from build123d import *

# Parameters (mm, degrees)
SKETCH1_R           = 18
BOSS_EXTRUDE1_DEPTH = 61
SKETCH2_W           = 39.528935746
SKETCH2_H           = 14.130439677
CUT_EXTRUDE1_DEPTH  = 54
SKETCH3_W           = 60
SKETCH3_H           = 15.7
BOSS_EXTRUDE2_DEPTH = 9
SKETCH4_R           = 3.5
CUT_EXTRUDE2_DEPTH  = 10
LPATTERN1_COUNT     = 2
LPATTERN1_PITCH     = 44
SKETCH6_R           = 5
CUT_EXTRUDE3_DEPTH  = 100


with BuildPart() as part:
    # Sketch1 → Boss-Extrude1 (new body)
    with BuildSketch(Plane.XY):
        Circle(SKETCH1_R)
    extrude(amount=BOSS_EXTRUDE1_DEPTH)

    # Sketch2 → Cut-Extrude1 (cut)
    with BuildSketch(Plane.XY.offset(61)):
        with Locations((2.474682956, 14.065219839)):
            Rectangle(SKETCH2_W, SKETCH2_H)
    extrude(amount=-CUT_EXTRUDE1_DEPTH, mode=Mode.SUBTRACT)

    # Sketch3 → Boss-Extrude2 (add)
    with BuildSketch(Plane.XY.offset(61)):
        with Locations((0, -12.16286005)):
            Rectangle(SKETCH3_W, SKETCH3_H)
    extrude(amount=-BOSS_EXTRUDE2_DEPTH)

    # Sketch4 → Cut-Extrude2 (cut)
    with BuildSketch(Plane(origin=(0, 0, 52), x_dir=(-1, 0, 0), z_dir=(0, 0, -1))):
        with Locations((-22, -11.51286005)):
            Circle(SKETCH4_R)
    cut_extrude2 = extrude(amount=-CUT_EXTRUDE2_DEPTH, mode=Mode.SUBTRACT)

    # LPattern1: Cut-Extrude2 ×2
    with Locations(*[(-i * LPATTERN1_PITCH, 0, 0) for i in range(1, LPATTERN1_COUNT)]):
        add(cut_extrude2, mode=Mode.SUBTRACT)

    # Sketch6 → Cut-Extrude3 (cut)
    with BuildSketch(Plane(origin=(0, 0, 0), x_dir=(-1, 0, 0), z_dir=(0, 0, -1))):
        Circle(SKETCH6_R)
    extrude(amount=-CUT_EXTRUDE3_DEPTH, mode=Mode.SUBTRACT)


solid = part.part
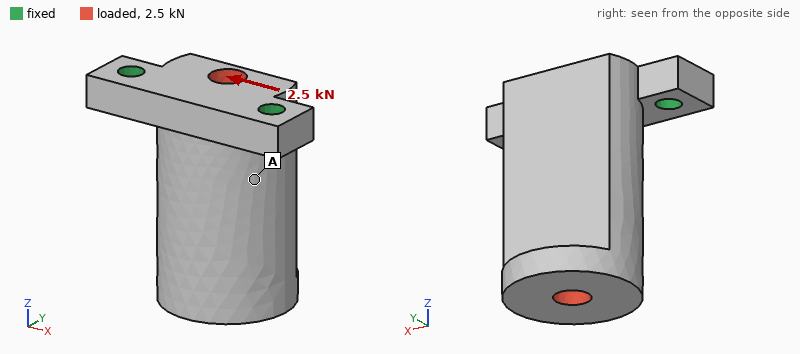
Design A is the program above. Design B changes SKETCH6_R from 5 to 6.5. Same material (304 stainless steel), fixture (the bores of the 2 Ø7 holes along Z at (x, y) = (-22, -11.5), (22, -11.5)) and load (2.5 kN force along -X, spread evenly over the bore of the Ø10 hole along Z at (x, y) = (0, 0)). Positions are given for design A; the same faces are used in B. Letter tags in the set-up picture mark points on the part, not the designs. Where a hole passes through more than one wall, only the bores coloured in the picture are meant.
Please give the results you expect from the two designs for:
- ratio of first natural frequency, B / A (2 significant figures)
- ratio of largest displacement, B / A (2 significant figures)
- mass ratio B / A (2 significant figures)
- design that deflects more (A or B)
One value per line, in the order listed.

1.0
1.1
0.93
B
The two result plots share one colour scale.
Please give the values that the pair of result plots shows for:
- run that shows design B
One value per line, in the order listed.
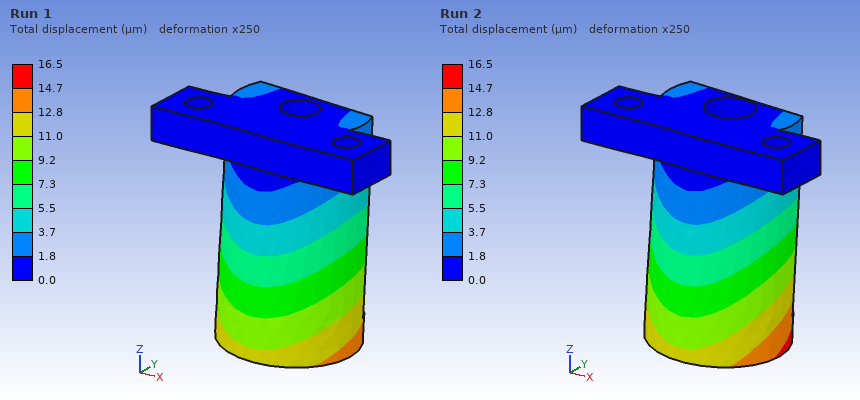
Run 2
